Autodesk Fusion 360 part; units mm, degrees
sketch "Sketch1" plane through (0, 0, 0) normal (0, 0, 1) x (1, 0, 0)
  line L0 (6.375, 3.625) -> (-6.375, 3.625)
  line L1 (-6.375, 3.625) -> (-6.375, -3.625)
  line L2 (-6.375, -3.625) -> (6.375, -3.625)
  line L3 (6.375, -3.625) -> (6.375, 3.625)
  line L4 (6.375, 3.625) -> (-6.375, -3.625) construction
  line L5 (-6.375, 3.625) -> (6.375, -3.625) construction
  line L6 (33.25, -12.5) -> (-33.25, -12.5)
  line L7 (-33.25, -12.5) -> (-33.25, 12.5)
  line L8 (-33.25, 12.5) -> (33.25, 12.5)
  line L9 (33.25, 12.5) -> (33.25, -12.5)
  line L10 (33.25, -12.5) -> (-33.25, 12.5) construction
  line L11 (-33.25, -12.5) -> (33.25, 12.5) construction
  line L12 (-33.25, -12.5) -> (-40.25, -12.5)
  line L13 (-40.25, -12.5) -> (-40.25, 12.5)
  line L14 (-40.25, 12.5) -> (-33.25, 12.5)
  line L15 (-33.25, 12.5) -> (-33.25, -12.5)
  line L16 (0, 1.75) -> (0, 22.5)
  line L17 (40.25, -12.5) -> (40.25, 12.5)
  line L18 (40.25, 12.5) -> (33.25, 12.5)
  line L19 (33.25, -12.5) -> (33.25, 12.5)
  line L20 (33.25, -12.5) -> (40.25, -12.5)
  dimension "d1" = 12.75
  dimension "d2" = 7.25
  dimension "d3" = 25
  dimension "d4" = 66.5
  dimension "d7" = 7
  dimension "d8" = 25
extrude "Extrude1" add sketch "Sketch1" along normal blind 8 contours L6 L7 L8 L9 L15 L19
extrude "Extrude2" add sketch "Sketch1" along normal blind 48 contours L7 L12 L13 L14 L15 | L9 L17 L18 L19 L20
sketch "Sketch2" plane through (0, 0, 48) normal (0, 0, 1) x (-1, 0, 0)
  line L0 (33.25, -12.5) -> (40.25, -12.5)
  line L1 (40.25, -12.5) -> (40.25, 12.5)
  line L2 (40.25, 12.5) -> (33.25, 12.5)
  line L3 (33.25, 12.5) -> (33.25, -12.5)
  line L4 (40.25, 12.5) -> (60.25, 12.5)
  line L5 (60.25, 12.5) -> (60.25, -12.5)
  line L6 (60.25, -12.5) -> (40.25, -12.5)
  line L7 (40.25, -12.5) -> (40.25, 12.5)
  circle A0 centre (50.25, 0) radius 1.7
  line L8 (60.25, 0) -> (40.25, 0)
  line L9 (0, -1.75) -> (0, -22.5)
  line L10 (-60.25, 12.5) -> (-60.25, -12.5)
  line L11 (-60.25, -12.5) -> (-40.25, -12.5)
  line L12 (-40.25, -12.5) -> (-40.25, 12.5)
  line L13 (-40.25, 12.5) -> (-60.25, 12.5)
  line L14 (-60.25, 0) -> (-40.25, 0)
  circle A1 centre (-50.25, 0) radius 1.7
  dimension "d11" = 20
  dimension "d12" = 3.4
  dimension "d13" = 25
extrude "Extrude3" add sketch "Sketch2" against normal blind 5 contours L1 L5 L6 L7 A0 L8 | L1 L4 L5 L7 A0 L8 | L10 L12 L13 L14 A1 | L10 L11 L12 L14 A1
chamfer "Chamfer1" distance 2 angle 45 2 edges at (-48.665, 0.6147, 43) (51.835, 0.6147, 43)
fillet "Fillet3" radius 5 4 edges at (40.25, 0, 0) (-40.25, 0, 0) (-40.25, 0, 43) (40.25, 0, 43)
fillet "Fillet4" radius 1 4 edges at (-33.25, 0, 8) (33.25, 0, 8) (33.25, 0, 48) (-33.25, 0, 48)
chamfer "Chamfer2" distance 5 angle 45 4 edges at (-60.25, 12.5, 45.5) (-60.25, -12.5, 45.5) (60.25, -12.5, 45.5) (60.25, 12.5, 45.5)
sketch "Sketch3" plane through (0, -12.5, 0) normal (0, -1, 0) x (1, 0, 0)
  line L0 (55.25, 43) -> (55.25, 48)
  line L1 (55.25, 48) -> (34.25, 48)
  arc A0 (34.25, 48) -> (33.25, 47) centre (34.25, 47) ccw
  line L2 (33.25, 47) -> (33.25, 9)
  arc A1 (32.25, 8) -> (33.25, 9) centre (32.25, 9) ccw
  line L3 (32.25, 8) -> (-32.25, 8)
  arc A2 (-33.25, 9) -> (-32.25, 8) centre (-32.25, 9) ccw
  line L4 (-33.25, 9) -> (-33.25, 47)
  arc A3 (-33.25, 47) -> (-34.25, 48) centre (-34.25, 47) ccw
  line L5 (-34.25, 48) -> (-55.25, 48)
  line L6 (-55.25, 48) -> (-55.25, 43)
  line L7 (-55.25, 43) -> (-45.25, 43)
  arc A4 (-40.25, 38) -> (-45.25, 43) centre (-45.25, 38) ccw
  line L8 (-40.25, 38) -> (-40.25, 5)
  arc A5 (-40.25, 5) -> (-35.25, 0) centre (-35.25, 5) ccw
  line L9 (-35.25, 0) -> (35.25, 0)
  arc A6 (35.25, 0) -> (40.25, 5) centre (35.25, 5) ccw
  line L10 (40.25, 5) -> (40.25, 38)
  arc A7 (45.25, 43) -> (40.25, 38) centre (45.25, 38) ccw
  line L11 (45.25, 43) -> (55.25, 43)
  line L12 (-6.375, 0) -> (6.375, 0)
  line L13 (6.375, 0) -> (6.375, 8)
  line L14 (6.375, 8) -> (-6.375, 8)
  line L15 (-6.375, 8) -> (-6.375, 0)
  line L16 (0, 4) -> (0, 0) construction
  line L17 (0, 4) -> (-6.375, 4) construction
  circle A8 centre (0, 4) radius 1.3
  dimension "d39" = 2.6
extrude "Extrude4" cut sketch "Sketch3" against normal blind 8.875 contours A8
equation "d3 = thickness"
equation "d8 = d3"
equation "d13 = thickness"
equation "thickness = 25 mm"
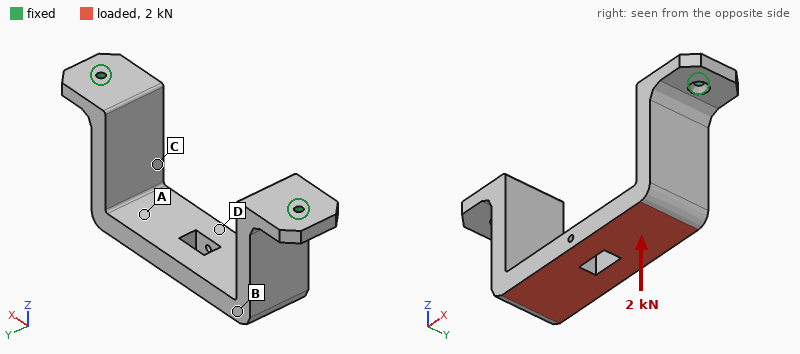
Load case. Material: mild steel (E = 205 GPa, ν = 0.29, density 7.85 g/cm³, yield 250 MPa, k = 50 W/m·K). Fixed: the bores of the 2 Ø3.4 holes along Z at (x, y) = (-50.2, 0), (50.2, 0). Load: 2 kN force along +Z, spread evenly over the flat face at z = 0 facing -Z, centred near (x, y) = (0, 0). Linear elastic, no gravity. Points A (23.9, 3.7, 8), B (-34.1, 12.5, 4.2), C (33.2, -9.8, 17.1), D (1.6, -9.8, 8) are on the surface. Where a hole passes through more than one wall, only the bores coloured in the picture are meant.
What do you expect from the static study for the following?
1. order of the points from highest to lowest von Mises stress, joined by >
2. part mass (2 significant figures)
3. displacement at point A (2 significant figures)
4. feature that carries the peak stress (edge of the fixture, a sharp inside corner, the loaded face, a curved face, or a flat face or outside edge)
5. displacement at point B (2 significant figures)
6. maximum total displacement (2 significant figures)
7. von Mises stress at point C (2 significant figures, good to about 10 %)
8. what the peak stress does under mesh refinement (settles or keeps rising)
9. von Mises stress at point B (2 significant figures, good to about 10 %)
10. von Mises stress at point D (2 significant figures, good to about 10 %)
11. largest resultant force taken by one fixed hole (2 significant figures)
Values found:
D > C > B > A
270 g
16 µm
edge of the fixture
8.8 µm
27 µm
27 MPa
keeps rising
15 MPa
35 MPa
1.1 kN
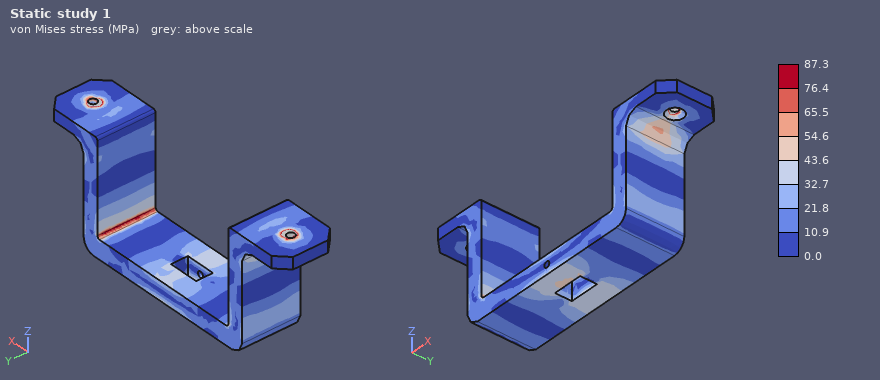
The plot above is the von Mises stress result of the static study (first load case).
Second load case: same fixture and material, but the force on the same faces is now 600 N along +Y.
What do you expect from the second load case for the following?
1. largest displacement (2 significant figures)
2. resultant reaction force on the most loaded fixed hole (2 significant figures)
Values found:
0.15 mm
300 N
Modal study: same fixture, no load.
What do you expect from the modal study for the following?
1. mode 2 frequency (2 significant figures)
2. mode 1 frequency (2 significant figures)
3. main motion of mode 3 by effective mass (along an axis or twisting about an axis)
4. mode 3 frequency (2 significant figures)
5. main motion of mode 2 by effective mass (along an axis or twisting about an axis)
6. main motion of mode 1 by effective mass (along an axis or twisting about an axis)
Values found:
1800 Hz
910 Hz
twisting about Z
2400 Hz
along X
along Y
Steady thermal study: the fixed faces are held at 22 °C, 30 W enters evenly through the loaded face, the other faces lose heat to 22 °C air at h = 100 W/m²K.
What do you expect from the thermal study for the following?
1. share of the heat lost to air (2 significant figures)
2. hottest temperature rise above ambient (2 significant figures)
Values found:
80 %
46 K
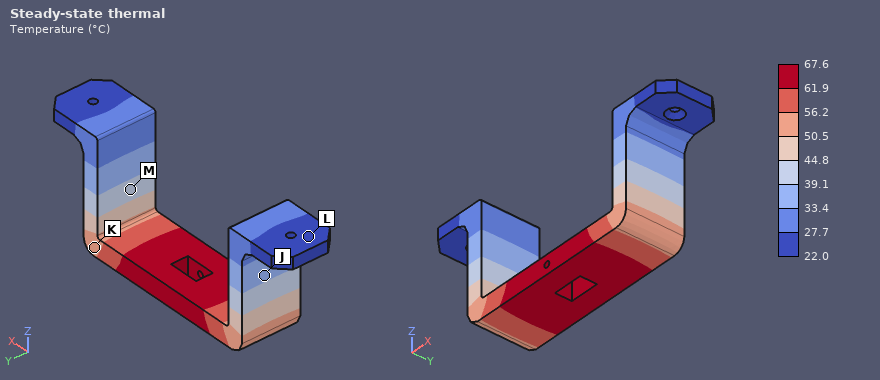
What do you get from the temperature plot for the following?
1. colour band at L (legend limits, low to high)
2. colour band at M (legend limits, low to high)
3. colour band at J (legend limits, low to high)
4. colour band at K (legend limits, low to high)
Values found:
22.0 to 27.7 °C
39.1 to 44.8 °C
33.4 to 39.1 °C
50.5 to 56.2 °C
